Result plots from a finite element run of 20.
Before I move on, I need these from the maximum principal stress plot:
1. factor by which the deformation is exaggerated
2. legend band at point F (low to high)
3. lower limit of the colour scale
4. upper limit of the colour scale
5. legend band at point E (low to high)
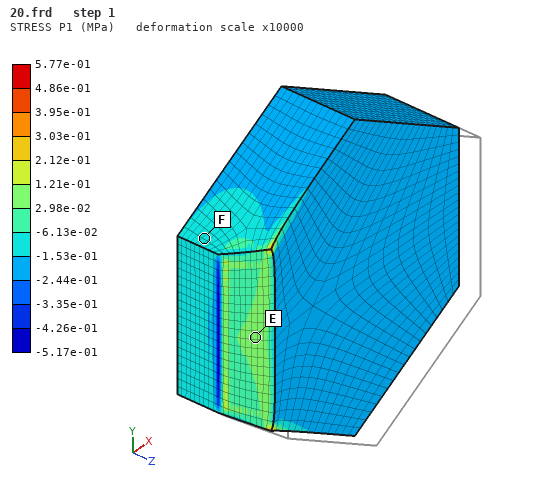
10000
-1.53e-01 to -6.13e-02 MPa
-5.17e-01 MPa
5.77e-01 MPa
2.98e-02 to 1.21e-01 MPa
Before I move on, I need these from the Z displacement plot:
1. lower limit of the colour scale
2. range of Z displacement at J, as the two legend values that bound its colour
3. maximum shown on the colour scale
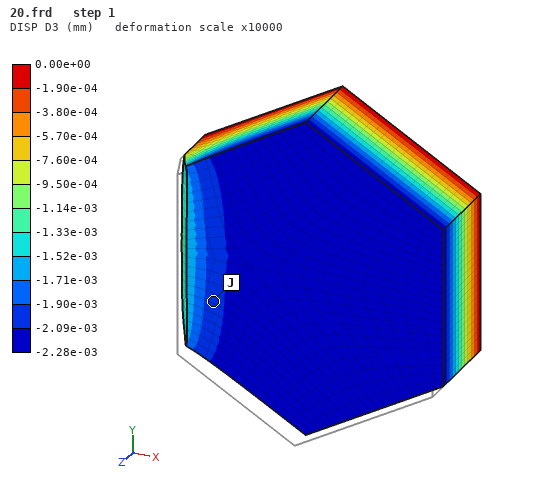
-2.28e-03 mm
-2.09e-03 to -1.90e-03 mm
0.00e+00 mm
